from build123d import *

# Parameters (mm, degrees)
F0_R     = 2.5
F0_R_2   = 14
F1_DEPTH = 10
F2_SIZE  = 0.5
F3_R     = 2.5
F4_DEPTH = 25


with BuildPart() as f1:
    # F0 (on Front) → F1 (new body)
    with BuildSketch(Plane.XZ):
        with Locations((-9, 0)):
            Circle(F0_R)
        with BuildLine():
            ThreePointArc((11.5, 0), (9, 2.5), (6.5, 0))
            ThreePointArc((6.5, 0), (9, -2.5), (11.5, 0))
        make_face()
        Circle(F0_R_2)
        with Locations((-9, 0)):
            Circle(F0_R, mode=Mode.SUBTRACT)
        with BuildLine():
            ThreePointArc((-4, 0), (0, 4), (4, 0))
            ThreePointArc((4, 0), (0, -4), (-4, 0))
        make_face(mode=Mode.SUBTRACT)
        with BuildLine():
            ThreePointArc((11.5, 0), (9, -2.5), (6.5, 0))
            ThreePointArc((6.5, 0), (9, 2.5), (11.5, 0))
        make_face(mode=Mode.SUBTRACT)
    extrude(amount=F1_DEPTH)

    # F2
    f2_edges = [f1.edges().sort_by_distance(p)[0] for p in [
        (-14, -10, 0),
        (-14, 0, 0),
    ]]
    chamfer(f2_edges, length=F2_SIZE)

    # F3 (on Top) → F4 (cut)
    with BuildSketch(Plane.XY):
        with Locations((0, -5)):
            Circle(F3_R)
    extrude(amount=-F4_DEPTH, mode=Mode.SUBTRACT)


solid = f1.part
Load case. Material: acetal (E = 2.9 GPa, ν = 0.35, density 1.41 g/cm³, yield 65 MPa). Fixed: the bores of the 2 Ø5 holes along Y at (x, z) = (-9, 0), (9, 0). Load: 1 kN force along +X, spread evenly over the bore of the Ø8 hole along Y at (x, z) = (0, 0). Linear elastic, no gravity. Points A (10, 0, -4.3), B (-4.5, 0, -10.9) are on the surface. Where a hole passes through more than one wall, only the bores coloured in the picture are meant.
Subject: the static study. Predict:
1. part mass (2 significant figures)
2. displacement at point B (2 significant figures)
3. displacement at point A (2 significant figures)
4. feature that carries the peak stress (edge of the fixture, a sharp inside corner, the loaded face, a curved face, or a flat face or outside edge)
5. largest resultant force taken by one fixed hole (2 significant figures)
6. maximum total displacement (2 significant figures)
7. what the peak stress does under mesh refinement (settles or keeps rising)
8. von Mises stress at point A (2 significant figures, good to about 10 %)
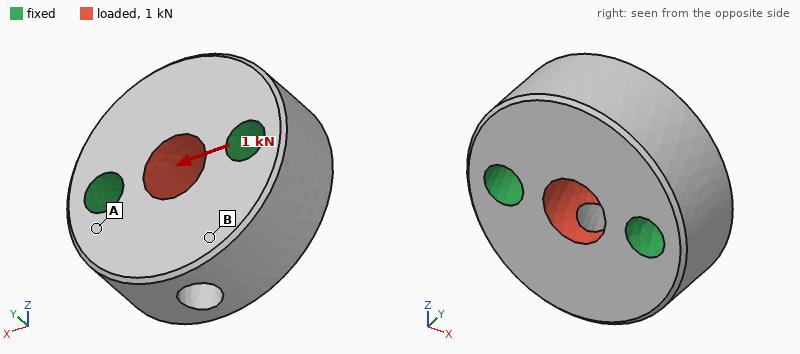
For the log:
7.1 g
5.8 µm
2.6 µm
edge of the fixture
500 N
14 µm
keeps rising
1.9 MPa
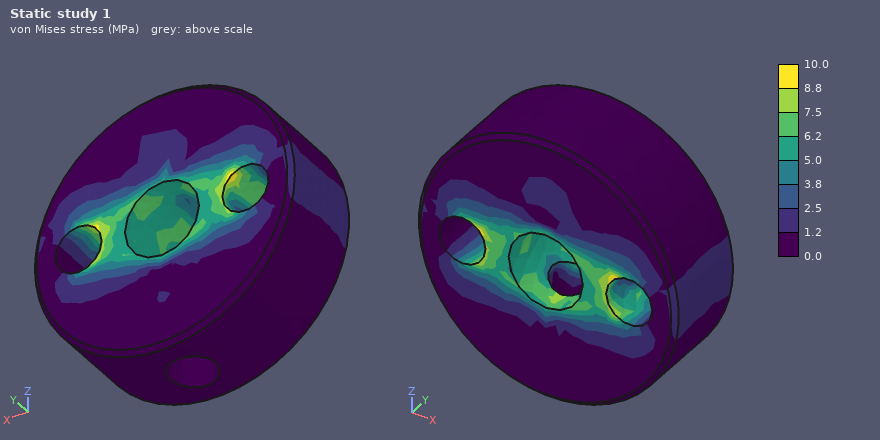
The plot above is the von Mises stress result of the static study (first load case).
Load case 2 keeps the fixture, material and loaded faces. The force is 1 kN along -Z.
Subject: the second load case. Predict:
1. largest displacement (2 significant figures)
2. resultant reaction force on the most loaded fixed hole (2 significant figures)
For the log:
19 µm
500 N
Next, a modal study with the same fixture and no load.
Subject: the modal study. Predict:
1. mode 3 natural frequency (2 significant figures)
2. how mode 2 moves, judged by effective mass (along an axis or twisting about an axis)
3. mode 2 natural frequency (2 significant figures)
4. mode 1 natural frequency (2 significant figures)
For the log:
16 kHz
along Y
12 kHz
11 kHz
